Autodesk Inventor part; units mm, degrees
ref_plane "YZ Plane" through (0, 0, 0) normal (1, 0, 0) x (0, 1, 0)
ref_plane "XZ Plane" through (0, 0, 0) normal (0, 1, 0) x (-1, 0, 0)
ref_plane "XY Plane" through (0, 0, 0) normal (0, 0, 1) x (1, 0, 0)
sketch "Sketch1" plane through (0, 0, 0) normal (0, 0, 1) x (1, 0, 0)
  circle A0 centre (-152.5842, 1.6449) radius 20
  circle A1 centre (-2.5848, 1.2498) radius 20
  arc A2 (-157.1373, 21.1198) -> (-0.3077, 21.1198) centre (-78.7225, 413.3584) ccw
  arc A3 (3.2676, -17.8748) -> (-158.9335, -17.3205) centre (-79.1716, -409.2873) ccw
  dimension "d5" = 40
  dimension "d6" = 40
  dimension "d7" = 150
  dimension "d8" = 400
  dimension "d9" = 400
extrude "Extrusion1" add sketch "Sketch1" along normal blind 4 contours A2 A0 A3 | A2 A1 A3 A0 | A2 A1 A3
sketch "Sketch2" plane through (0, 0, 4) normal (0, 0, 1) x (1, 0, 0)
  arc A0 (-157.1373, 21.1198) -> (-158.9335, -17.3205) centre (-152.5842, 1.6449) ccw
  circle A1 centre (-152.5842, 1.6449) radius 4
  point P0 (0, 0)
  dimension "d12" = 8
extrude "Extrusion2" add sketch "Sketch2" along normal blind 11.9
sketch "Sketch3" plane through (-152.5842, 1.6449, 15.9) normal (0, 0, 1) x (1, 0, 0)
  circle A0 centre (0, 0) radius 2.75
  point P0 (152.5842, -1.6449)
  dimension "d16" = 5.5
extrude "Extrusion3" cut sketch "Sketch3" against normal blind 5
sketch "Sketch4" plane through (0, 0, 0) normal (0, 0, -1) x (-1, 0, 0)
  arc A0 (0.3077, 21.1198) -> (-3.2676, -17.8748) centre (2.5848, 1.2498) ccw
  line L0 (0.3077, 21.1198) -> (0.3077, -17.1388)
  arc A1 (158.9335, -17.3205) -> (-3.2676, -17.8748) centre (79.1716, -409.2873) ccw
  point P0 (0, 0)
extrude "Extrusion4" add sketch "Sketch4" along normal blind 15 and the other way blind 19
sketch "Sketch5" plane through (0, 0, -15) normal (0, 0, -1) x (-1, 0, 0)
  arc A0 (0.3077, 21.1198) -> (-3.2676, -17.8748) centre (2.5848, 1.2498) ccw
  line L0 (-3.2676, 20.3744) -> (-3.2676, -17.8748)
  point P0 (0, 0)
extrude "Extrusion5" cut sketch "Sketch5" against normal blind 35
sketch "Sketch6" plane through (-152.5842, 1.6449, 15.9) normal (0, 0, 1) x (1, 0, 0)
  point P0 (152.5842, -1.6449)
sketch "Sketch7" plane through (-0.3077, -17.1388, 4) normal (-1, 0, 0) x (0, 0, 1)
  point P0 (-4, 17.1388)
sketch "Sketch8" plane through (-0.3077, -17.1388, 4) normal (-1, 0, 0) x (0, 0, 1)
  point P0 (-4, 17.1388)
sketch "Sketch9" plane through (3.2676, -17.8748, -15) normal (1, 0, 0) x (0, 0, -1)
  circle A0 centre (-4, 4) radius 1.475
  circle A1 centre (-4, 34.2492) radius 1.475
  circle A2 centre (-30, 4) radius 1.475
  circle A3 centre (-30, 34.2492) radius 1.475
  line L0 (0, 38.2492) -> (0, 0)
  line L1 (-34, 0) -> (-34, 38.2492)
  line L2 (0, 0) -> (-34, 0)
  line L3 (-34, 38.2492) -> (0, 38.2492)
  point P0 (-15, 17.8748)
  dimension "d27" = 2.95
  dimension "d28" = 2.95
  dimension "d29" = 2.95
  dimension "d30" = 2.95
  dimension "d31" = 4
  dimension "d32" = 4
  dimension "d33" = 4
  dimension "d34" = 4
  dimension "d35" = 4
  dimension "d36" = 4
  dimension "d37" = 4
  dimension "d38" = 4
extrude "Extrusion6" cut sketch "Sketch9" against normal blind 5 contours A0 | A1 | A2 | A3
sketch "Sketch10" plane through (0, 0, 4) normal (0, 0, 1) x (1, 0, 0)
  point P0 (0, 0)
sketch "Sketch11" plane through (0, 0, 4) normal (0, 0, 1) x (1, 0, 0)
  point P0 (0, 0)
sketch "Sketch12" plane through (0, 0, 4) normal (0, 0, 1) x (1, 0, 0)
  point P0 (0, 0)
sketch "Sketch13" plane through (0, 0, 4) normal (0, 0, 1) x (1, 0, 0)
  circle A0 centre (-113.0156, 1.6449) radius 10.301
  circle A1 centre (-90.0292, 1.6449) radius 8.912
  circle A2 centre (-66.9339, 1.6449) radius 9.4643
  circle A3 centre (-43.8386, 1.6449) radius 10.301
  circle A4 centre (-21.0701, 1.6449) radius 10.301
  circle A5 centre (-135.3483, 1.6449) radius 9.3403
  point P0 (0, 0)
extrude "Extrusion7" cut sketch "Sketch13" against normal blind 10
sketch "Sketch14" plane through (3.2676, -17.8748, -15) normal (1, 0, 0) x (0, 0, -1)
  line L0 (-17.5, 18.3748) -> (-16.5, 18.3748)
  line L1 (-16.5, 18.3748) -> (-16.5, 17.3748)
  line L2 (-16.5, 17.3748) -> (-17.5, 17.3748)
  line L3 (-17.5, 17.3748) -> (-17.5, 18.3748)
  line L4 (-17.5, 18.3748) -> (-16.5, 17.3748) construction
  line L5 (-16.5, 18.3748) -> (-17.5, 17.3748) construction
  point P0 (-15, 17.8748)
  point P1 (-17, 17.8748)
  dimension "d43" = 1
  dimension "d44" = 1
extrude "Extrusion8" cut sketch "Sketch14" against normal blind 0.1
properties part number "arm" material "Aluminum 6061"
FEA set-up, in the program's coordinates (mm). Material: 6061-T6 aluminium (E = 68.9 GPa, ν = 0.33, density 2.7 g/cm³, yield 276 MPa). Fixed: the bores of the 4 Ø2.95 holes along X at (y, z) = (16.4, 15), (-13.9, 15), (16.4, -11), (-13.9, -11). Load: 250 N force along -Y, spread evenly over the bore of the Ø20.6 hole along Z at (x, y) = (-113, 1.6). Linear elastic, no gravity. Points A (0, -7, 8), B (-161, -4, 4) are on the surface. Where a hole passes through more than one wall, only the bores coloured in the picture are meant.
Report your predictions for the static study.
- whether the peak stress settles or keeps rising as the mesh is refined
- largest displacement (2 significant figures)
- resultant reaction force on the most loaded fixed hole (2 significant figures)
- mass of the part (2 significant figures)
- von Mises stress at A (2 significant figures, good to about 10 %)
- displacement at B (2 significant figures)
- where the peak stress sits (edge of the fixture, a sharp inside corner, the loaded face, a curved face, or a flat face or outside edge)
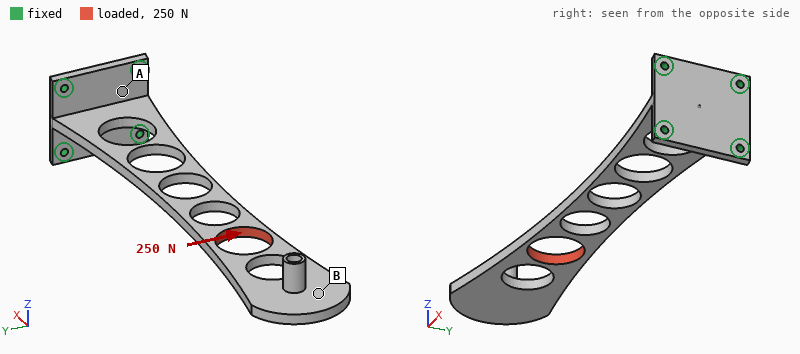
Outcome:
keeps rising
1.2 mm
490 N
46 g
32 MPa
1.1 mm
edge of the fixture
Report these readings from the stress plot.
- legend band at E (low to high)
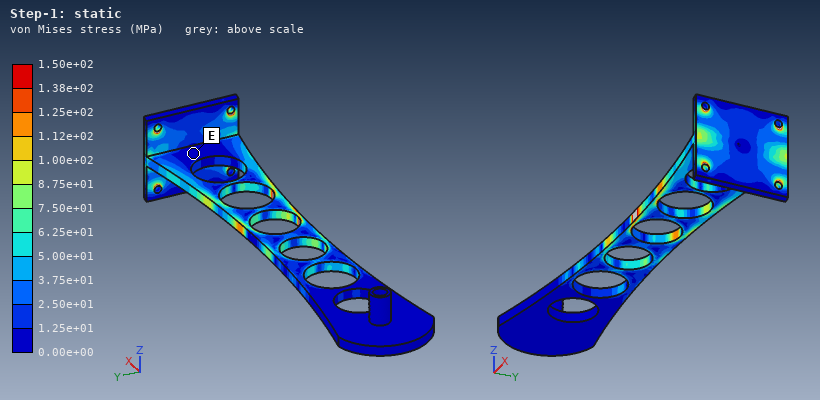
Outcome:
0.00e+00 to 1.25e+01 MPa
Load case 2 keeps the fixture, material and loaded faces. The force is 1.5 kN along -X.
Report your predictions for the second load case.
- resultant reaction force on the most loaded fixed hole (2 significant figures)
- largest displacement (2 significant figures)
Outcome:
390 N
0.18 mm
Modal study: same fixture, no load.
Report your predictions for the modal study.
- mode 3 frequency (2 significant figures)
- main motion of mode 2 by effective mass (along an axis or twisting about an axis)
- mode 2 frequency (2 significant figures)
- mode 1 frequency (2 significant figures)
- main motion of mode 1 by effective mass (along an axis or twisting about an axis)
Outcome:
580 Hz
along Y
490 Hz
70 Hz
along Z
